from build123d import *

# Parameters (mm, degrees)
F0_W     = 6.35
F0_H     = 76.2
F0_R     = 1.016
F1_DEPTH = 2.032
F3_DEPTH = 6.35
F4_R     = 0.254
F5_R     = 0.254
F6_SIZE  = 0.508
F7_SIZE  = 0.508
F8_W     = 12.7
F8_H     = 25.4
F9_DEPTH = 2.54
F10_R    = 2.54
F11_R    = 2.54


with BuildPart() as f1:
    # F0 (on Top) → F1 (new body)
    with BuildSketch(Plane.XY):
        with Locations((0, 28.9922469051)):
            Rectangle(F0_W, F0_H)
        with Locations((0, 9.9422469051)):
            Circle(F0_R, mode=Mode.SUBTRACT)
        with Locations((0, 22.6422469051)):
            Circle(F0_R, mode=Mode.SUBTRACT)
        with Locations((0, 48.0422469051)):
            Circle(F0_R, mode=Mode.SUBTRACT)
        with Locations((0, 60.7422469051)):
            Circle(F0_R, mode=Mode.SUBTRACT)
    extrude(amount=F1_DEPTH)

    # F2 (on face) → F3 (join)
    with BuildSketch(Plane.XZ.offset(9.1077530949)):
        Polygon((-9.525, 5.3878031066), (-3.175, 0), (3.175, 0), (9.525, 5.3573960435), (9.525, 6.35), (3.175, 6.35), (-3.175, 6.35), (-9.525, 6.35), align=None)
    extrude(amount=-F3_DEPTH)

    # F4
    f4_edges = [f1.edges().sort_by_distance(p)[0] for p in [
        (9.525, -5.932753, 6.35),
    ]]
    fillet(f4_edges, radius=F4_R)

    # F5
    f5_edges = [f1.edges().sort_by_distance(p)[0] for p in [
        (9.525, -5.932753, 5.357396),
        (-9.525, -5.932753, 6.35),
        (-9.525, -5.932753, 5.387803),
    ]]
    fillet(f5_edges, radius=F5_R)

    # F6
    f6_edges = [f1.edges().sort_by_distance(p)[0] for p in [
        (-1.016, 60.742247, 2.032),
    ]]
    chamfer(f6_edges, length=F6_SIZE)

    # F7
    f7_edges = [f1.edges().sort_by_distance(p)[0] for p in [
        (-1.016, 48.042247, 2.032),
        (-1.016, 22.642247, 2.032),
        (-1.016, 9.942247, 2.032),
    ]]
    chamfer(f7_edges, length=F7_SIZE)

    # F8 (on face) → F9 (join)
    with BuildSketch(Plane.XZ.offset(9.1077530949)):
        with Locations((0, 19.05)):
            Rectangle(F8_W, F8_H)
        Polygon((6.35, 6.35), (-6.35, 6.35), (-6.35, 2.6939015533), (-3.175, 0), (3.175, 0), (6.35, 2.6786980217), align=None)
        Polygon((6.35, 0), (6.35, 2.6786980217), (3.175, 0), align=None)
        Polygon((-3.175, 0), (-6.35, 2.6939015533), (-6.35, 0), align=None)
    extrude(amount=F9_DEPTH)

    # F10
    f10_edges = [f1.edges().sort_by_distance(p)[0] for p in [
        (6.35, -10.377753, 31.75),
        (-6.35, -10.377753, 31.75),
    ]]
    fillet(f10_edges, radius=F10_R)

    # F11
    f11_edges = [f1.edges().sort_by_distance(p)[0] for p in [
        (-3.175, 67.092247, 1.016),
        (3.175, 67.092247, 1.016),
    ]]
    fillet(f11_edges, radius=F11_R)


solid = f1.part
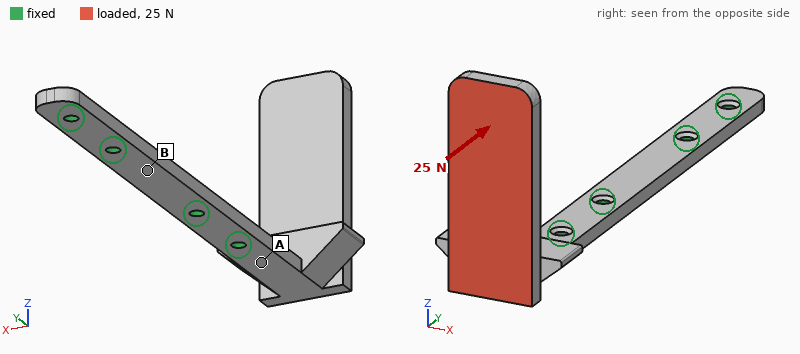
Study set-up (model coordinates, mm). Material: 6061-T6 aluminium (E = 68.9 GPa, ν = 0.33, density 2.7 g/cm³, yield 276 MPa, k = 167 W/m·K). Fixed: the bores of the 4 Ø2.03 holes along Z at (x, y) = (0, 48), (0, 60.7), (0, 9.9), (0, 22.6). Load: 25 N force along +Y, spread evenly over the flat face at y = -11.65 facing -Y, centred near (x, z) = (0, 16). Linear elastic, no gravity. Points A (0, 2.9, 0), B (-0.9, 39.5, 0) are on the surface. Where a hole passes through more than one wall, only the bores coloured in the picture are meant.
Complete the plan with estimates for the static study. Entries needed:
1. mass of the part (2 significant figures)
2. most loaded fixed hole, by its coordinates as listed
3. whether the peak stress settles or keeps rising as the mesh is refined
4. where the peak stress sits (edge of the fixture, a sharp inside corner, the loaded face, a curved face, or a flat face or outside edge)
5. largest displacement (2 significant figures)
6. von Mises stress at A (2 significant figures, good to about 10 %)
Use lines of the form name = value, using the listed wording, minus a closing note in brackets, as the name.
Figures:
mass of the part = 6.6 g
most loaded fixed hole, by its coordinates as listed = (0, 9.9)
whether the peak stress settles or keeps rising as the mesh is refined = keeps rising
where the peak stress sits = edge of the fixture
largest displacement = 0.60 mm
von Mises stress at A = 81 MPa
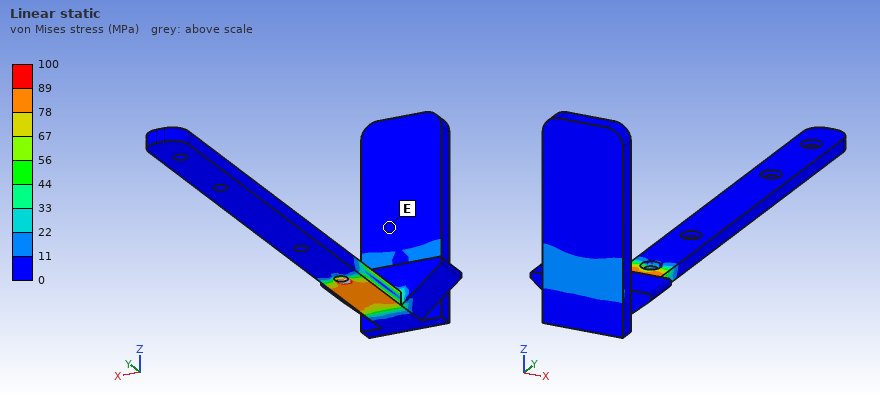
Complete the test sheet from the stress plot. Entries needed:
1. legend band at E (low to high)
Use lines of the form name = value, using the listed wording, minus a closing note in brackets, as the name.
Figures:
legend band at E = 0 to 11 MPa
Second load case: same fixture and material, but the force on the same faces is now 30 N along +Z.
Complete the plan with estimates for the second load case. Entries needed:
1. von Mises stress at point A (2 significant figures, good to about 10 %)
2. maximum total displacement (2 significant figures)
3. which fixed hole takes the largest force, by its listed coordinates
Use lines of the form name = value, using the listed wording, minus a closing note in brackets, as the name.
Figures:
von Mises stress at point A = 98 MPa
maximum total displacement = 0.69 mm
which fixed hole takes the largest force, by its listed coordinates = (0, 9.9)
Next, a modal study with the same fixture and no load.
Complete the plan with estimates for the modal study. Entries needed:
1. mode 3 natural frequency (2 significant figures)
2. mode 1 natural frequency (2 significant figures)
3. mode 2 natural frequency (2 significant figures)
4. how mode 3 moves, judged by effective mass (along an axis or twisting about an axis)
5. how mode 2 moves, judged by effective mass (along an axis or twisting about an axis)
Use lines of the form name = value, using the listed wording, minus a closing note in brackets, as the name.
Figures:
mode 3 natural frequency = 2900 Hz
mode 1 natural frequency = 610 Hz
mode 2 natural frequency = 880 Hz
how mode 3 moves, judged by effective mass = along Z
how mode 2 moves, judged by effective mass = along X
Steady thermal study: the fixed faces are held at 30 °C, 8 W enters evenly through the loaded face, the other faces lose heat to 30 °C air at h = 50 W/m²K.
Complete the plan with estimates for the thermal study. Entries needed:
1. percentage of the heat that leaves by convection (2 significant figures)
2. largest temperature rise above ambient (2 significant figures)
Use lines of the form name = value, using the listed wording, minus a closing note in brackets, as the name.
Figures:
percentage of the heat that leaves by convection = 28 %
largest temperature rise above ambient = 54 K
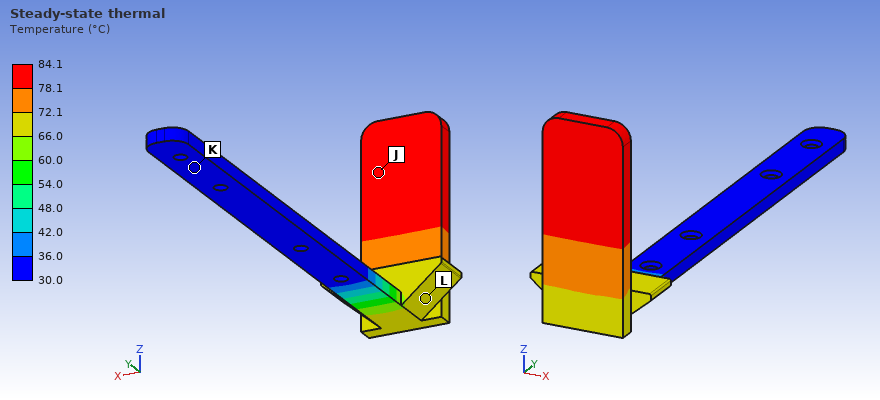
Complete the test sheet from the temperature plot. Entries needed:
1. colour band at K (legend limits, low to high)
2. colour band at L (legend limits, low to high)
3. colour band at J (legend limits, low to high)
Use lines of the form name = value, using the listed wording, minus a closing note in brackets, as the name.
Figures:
colour band at K = 30.0 to 36.0 °C
colour band at L = 66.0 to 72.1 °C
colour band at J = 78.1 to 84.1 °C
